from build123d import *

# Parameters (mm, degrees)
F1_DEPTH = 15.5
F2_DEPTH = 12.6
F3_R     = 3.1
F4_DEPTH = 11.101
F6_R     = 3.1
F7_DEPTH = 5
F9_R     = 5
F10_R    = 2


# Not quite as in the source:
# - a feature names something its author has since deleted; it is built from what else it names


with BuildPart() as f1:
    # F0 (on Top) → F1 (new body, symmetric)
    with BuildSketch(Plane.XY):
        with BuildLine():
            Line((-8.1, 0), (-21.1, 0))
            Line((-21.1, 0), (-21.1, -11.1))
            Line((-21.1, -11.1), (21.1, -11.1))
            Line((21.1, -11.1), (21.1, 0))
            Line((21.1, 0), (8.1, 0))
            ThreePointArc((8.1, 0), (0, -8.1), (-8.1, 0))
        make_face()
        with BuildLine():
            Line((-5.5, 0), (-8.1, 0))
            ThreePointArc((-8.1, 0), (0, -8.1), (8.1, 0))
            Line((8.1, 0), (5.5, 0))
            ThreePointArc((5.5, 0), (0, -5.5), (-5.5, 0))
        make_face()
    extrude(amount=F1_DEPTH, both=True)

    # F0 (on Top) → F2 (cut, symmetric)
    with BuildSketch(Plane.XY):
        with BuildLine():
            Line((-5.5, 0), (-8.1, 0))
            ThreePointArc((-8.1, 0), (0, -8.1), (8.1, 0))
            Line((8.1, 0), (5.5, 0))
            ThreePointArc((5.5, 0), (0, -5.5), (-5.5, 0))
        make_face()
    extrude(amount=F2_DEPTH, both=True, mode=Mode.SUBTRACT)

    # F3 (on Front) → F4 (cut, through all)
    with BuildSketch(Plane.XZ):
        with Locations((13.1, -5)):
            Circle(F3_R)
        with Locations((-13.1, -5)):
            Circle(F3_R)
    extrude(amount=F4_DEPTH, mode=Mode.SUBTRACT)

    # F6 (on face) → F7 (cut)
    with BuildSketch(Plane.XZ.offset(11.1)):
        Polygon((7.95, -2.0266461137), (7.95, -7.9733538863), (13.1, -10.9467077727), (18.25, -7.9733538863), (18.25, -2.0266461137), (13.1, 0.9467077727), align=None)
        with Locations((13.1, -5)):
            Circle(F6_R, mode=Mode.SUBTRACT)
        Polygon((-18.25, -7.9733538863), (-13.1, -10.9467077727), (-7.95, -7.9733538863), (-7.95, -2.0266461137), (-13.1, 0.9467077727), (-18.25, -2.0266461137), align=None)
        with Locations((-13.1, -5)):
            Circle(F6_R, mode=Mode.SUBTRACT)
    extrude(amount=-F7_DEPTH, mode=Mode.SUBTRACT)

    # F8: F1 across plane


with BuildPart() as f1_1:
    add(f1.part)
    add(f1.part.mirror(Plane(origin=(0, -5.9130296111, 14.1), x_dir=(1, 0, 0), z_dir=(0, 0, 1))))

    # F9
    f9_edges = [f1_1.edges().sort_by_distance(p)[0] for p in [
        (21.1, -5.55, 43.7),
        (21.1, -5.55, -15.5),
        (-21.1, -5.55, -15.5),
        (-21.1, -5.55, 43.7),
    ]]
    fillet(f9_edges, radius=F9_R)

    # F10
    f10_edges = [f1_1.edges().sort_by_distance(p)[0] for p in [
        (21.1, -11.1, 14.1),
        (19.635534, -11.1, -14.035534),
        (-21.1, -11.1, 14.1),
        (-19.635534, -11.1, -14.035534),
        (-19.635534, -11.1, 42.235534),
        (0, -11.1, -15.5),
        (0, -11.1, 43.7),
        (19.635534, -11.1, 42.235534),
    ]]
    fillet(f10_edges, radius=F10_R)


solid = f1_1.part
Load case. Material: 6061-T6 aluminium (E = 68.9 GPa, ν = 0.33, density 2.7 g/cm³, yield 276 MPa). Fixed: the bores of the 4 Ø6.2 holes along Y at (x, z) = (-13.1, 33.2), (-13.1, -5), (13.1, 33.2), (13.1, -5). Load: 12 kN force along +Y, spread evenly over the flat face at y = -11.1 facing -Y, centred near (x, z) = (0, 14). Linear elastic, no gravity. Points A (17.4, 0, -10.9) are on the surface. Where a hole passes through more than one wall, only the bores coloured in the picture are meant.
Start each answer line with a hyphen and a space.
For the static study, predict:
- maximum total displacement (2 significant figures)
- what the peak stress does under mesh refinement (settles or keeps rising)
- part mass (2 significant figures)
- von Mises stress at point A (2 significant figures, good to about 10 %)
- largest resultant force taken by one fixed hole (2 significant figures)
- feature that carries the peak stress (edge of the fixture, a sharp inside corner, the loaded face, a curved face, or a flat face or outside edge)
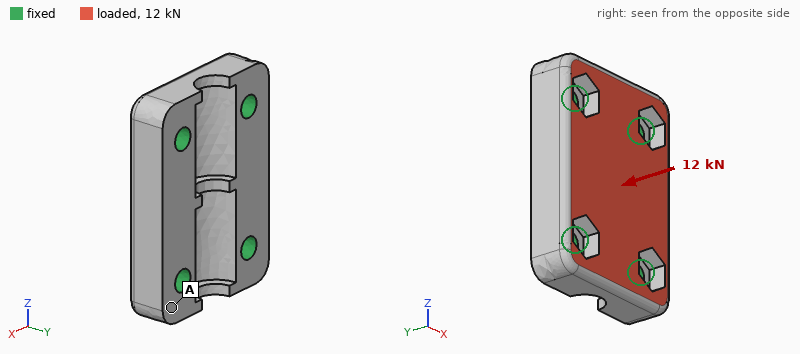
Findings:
- 22 µm
- keeps rising
- 52 g
- 12 MPa
- 3.4 kN
- edge of the fixture
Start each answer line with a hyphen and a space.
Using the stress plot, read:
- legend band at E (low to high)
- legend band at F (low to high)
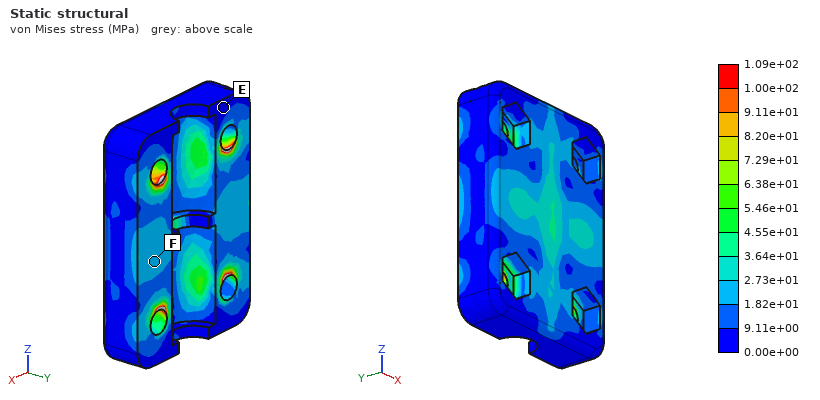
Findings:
- 0.00e+00 to 9.11e+00 MPa
- 1.82e+01 to 2.73e+01 MPa
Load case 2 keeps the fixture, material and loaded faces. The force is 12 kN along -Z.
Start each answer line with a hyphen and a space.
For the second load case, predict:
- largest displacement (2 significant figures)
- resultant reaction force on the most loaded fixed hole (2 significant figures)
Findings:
- 14 µm
- 3.2 kN
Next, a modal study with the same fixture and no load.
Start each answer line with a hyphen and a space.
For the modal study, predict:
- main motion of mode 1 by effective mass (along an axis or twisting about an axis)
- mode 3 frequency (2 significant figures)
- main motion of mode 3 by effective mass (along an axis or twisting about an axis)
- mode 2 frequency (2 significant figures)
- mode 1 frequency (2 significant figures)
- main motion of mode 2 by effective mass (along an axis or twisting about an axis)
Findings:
- along Y
- 28 kHz
- along X
- 25 kHz
- 23 kHz
- twisting about Z
